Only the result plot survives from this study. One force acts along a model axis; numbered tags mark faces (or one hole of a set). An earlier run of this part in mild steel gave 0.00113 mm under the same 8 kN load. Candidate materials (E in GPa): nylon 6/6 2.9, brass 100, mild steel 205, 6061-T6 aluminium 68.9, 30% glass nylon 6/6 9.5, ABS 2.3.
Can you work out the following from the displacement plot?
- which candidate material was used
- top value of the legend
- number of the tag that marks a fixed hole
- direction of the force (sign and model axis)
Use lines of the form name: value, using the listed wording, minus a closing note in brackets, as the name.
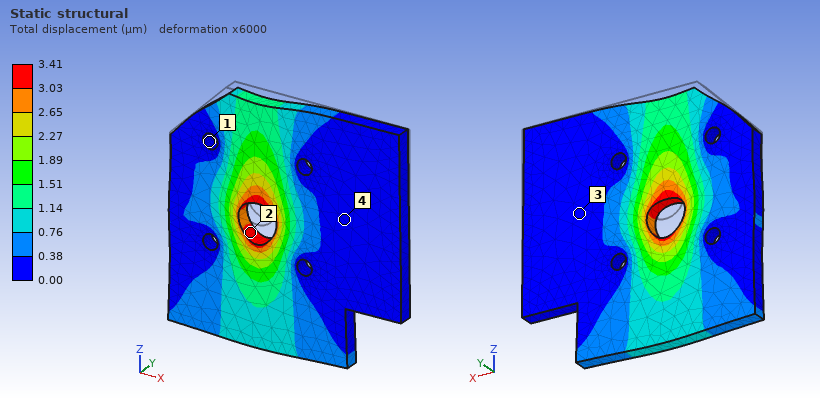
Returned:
which candidate material was used: 6061-T6 aluminium
top value of the legend: 3.41 µm
number of the tag that marks a fixed hole: 1
direction of the force: -Z
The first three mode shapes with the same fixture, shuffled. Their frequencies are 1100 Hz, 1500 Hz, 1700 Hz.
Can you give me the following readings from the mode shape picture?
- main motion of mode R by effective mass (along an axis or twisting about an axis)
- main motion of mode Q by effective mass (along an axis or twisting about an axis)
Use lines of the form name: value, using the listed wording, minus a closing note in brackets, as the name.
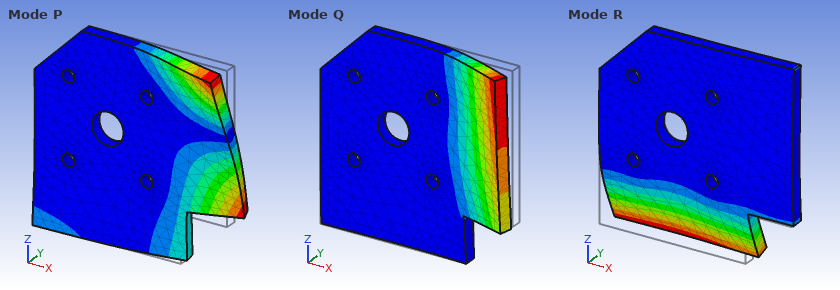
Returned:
main motion of mode R by effective mass: along Y
main motion of mode Q by effective mass: along Y
